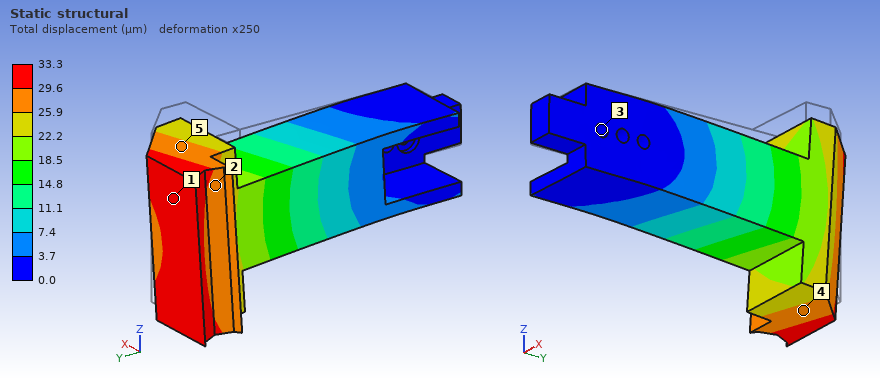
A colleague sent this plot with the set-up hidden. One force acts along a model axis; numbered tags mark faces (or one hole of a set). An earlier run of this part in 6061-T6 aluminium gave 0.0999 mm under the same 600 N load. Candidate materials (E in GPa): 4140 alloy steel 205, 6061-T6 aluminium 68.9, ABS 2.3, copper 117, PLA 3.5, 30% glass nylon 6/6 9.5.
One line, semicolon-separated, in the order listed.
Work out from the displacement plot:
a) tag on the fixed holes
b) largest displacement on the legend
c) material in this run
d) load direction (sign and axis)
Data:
3; 33.3 µm; 4140 alloy steel; -Z
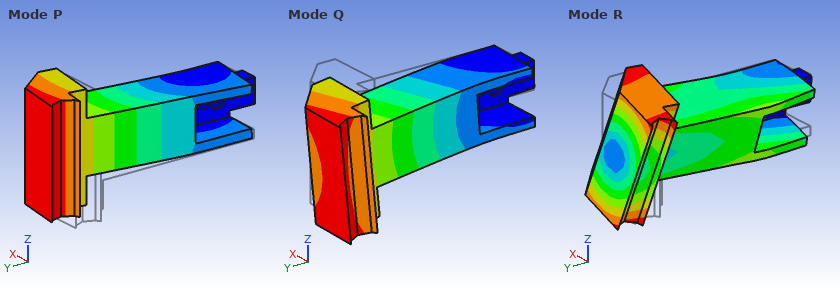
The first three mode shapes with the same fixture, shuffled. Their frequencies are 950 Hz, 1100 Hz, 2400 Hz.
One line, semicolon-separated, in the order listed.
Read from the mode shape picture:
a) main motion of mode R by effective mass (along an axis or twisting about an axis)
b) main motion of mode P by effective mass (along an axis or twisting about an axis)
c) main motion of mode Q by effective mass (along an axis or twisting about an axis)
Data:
twisting about Y; along X; along Z
